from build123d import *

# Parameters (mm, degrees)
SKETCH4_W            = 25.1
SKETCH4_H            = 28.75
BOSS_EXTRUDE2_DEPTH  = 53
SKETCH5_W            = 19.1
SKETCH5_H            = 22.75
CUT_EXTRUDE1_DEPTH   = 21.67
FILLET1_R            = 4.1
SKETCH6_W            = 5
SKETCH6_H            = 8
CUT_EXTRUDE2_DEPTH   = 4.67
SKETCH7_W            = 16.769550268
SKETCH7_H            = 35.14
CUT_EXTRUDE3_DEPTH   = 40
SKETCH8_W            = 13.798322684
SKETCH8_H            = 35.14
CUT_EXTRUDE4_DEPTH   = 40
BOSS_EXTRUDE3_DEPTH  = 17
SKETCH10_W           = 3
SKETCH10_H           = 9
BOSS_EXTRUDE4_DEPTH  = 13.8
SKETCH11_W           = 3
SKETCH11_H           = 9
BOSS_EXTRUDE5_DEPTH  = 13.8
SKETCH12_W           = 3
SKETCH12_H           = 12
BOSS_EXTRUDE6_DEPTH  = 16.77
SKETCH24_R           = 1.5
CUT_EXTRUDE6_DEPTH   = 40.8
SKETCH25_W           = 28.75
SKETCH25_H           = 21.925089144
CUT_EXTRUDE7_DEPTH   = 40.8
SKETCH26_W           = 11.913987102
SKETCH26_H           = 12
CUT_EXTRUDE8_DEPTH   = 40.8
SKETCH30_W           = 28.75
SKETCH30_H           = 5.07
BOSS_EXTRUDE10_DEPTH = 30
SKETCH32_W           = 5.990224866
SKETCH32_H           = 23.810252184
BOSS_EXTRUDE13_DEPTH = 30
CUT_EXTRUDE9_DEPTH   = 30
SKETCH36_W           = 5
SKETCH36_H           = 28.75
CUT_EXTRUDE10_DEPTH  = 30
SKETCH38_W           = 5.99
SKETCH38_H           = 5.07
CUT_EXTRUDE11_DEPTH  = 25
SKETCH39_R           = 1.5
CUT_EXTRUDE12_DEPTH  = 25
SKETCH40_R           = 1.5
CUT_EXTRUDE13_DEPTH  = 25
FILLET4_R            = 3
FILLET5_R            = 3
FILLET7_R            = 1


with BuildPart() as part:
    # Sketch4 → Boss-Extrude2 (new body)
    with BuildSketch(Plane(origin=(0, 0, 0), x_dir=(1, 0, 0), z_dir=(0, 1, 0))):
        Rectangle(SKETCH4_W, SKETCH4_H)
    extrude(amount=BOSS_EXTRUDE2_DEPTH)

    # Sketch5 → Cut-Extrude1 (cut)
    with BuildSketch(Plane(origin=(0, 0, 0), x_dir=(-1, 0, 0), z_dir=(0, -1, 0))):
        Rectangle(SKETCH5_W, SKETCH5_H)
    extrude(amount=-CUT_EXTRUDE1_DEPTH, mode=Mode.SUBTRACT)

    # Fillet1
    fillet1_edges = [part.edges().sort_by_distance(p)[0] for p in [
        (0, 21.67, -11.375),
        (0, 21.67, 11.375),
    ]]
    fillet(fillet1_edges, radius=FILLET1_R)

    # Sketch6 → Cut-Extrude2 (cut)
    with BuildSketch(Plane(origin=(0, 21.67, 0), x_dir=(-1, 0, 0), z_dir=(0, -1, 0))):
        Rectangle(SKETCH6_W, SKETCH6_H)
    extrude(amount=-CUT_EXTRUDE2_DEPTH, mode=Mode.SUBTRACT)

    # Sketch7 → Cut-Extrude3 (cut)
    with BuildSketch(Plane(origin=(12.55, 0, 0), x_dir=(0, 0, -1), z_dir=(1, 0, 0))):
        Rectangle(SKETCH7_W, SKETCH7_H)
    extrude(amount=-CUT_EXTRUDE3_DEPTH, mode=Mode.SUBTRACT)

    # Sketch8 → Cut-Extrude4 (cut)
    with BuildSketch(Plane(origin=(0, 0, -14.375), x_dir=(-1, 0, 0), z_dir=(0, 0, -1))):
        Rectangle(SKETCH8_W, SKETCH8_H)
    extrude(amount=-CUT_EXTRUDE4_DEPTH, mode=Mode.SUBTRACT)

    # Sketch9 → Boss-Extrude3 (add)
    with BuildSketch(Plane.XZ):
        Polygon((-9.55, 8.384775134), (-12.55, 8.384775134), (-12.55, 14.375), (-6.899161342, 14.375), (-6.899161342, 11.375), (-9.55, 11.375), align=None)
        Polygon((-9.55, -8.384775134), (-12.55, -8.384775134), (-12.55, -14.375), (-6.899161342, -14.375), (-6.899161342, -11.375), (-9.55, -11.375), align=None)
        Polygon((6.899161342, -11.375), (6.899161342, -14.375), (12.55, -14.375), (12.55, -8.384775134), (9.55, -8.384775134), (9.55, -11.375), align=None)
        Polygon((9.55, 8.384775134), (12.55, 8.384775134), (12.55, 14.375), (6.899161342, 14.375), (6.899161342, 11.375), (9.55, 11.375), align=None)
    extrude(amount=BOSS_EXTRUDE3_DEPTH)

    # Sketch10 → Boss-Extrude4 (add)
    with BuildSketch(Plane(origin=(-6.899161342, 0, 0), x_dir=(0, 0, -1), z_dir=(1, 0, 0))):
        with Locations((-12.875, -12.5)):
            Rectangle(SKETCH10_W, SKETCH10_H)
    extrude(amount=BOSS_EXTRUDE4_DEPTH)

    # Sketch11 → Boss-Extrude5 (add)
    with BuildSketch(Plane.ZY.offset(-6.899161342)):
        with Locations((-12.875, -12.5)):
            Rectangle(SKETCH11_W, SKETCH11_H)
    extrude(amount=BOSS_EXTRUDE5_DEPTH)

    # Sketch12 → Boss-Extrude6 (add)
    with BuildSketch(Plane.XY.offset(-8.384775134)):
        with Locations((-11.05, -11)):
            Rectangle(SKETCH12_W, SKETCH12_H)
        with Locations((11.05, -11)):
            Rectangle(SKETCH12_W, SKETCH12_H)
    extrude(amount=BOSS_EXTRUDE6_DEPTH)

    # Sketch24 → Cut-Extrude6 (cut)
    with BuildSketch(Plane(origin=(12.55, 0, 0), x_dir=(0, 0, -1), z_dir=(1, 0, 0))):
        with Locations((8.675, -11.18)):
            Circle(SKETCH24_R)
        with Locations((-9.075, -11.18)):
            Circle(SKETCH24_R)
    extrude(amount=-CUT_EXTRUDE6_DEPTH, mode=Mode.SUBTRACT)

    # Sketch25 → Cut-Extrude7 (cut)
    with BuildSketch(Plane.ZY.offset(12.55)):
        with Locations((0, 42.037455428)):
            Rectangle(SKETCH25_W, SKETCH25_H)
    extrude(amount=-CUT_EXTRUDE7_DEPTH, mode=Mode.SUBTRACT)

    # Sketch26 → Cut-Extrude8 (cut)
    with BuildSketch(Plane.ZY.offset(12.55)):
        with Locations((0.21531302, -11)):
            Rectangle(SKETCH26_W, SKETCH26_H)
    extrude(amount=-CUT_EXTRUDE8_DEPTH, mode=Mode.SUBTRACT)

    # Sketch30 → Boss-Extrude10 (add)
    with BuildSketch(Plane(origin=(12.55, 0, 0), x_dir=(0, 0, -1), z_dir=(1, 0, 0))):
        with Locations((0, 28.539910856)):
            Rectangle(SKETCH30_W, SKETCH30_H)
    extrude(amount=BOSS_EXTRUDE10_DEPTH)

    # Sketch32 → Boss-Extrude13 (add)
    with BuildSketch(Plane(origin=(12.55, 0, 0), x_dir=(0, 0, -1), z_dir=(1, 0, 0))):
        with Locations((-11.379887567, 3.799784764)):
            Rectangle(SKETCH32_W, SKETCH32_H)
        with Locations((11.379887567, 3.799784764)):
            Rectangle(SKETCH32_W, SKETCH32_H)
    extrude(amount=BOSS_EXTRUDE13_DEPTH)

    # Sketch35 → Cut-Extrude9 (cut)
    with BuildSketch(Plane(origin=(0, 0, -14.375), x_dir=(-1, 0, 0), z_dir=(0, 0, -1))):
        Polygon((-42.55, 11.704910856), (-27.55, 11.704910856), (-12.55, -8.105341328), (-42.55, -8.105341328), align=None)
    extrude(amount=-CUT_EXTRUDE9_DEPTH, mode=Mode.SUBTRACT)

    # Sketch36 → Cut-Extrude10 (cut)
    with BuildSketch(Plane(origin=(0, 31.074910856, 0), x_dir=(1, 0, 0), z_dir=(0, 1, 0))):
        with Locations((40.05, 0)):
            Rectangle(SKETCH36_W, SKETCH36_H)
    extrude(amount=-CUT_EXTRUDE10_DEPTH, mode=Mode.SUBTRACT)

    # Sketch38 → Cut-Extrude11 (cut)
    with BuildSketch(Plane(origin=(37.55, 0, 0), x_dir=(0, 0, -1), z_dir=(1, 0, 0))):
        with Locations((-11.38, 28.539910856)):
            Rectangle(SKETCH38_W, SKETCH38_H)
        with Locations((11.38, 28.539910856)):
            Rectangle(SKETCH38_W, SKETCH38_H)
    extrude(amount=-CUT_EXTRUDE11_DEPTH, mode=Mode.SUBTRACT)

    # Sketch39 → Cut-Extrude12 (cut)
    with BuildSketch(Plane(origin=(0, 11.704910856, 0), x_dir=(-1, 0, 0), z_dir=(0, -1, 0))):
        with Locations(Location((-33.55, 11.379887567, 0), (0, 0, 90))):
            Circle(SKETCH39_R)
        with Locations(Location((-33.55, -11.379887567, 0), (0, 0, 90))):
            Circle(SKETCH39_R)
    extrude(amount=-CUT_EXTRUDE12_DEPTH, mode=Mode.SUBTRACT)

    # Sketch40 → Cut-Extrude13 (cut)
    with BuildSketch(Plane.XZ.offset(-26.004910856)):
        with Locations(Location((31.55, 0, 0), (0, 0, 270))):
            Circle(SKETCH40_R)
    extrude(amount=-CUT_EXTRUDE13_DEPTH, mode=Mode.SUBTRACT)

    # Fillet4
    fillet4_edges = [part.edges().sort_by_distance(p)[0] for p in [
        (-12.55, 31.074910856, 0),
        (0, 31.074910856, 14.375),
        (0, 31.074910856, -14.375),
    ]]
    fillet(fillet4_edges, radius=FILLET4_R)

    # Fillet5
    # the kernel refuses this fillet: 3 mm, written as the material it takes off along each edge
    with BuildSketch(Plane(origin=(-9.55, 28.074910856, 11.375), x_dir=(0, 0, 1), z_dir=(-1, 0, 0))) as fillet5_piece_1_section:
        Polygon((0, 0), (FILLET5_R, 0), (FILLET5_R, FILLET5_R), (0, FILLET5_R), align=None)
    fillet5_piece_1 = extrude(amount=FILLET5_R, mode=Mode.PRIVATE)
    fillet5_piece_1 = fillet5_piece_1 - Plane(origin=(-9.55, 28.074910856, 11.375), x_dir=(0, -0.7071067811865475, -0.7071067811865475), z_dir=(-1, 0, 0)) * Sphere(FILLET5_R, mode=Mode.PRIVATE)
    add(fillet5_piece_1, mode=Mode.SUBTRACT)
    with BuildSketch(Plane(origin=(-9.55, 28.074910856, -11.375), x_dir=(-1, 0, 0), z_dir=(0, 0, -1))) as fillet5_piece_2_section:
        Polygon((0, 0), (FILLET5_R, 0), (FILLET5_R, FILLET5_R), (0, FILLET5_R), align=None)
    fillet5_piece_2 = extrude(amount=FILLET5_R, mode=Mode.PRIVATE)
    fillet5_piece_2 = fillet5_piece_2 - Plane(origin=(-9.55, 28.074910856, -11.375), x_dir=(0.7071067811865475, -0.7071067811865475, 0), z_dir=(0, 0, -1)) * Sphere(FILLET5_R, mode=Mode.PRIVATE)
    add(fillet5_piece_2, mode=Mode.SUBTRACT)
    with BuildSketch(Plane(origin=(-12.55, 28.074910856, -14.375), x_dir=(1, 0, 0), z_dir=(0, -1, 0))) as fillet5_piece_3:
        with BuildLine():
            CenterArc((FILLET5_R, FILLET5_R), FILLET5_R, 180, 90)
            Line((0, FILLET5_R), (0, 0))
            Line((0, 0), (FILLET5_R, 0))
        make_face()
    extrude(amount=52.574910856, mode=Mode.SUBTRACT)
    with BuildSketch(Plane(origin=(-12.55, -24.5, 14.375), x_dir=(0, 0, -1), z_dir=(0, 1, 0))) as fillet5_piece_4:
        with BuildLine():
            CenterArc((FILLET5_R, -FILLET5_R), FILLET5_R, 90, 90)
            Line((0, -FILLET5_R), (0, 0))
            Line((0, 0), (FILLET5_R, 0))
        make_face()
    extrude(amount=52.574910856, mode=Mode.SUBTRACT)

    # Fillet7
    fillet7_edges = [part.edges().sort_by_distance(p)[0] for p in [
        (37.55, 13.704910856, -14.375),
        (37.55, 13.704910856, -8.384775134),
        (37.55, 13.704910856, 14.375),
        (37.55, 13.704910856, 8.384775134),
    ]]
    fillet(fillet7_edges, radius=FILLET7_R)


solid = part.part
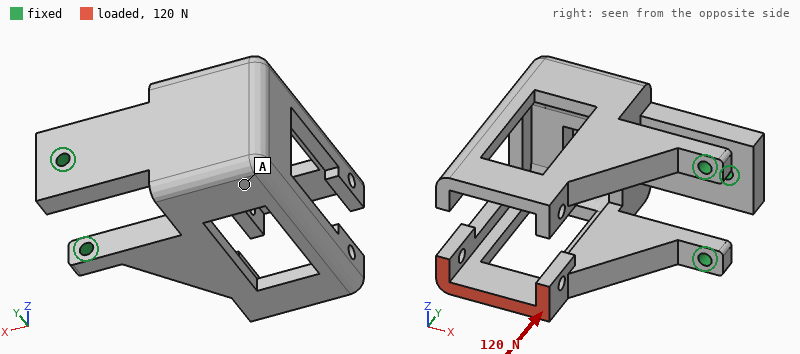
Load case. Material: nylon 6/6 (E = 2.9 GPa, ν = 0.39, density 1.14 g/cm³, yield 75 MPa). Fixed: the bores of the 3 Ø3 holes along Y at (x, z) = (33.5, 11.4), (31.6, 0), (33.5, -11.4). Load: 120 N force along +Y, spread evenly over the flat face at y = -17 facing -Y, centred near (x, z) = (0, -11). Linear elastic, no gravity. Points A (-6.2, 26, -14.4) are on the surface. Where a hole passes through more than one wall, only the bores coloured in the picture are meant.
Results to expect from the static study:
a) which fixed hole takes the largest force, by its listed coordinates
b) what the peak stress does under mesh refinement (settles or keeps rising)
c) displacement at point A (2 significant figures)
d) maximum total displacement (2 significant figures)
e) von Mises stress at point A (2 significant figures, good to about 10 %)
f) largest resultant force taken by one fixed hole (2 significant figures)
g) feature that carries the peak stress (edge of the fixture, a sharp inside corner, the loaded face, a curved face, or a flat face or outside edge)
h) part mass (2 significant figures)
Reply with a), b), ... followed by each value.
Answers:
a) (31.6, 0)
b) keeps rising
c) 0.45 mm
d) 0.86 mm
e) 2.5 MPa
f) 190 N
g) edge of the fixture
h) 20 g
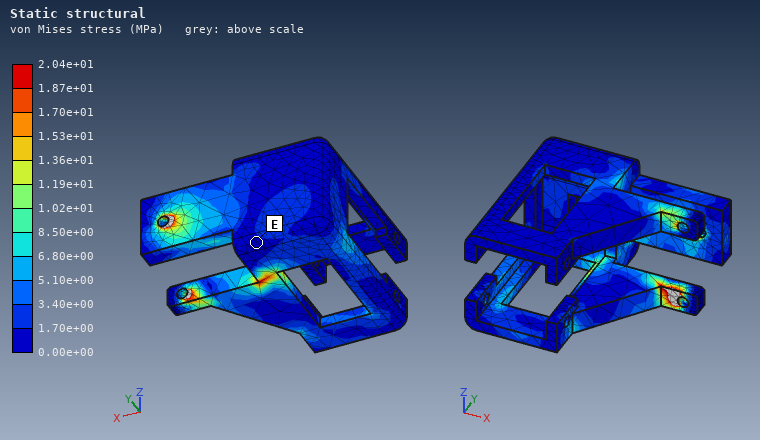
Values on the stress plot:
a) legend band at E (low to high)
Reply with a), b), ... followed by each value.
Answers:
a) 0.00e+00 to 1.70e+00 MPa
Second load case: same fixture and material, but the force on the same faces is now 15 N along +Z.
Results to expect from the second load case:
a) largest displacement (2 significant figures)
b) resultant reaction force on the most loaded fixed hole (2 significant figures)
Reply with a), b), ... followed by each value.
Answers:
a) 0.88 mm
b) 10 N
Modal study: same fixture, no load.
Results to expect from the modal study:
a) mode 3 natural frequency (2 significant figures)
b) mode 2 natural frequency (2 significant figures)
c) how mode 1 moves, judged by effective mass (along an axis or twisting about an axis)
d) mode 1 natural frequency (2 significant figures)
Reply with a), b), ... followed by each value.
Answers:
a) 860 Hz
b) 830 Hz
c) along Z
d) 490 Hz
